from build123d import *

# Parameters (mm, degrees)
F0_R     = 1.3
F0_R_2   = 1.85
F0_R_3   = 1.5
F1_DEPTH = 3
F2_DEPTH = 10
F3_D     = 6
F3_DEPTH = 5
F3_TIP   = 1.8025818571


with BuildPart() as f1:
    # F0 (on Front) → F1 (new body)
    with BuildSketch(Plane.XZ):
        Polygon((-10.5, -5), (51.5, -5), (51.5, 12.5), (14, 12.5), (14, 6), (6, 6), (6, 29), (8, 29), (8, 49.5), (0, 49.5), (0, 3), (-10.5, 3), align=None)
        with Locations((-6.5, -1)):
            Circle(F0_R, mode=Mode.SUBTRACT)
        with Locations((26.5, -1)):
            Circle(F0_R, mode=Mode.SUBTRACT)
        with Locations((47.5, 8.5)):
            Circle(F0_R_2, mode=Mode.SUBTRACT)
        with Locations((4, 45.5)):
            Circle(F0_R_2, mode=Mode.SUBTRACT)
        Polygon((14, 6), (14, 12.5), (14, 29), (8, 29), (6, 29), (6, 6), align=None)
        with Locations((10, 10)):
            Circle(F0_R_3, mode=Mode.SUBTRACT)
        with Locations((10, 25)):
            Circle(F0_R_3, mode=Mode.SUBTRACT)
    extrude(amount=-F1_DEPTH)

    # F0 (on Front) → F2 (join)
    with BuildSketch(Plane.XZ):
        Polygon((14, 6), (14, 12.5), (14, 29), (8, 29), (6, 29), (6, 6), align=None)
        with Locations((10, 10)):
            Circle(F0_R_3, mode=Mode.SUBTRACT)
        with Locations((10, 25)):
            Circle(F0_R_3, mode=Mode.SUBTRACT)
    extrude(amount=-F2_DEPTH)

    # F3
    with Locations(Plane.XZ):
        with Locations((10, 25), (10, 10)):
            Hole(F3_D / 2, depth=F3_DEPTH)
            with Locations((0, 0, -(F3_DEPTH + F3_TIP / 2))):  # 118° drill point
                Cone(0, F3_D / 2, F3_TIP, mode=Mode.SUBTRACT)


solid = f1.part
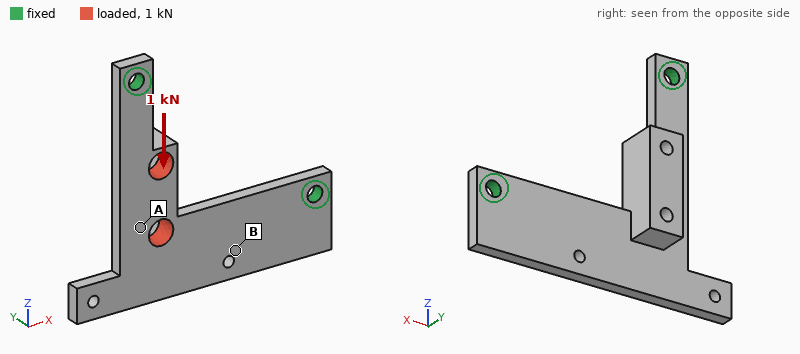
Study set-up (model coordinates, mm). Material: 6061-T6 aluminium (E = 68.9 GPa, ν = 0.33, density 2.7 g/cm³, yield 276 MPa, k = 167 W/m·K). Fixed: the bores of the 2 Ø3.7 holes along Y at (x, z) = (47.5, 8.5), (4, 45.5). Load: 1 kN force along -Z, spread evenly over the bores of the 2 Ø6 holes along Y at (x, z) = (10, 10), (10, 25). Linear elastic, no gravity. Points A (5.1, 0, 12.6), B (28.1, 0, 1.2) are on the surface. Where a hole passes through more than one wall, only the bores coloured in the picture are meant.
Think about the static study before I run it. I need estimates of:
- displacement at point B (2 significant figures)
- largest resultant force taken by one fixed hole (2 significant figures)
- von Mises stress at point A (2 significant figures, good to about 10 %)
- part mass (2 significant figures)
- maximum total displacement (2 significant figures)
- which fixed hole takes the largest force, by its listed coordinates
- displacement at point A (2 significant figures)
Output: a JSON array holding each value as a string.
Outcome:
["0.038 mm", "900 N", "22 MPa", "13 g", "0.17 mm", "(4, 45.5)", "0.073 mm"]
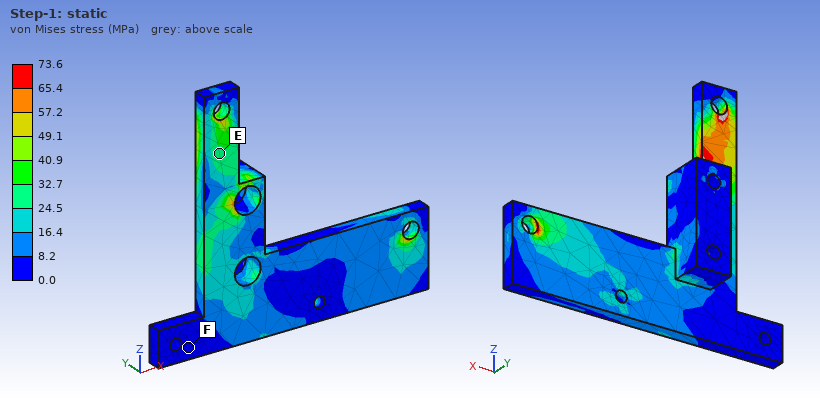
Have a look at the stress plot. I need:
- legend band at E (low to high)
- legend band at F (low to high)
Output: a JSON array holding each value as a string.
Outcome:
["24.5 to 32.7 MPa", "0.0 to 8.2 MPa"]
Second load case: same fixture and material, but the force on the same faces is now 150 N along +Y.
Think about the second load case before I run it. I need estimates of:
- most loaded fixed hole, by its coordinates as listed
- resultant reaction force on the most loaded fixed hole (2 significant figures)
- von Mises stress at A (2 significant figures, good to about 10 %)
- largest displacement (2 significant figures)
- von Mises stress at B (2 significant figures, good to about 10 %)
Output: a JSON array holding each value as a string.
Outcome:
["(4, 45.5)", "93 N", "12 MPa", "0.37 mm", "16 MPa"]
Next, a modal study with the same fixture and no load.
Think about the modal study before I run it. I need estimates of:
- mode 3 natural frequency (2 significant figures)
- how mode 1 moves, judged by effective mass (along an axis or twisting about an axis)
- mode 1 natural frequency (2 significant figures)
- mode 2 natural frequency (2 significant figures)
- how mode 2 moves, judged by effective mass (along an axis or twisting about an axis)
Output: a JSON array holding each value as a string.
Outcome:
["6200 Hz", "along Y", "1200 Hz", "4400 Hz", "along Y"]
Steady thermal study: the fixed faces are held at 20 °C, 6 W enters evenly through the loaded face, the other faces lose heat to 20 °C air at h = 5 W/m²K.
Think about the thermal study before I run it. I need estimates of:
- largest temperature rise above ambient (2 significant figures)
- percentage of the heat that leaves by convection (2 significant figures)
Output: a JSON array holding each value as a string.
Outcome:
["16 K", "3.1 %"]
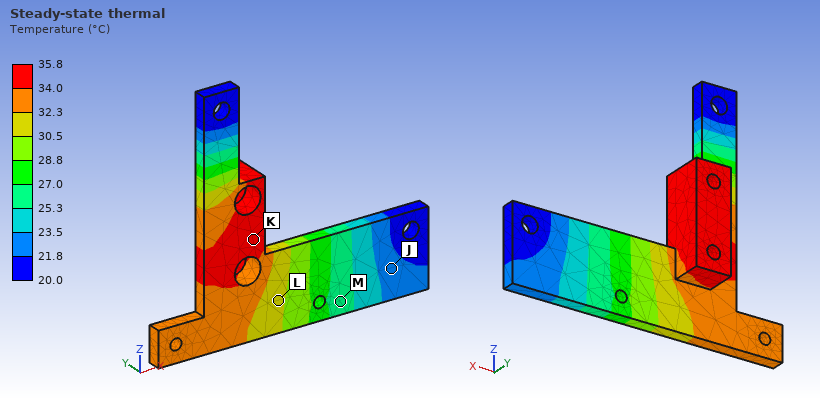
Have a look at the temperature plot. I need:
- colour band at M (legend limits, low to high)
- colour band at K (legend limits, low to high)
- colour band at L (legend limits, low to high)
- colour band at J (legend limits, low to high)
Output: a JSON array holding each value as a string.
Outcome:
["25.3 to 27.0 °C", "34.0 to 35.8 °C", "30.5 to 32.3 °C", "21.8 to 23.5 °C"]
